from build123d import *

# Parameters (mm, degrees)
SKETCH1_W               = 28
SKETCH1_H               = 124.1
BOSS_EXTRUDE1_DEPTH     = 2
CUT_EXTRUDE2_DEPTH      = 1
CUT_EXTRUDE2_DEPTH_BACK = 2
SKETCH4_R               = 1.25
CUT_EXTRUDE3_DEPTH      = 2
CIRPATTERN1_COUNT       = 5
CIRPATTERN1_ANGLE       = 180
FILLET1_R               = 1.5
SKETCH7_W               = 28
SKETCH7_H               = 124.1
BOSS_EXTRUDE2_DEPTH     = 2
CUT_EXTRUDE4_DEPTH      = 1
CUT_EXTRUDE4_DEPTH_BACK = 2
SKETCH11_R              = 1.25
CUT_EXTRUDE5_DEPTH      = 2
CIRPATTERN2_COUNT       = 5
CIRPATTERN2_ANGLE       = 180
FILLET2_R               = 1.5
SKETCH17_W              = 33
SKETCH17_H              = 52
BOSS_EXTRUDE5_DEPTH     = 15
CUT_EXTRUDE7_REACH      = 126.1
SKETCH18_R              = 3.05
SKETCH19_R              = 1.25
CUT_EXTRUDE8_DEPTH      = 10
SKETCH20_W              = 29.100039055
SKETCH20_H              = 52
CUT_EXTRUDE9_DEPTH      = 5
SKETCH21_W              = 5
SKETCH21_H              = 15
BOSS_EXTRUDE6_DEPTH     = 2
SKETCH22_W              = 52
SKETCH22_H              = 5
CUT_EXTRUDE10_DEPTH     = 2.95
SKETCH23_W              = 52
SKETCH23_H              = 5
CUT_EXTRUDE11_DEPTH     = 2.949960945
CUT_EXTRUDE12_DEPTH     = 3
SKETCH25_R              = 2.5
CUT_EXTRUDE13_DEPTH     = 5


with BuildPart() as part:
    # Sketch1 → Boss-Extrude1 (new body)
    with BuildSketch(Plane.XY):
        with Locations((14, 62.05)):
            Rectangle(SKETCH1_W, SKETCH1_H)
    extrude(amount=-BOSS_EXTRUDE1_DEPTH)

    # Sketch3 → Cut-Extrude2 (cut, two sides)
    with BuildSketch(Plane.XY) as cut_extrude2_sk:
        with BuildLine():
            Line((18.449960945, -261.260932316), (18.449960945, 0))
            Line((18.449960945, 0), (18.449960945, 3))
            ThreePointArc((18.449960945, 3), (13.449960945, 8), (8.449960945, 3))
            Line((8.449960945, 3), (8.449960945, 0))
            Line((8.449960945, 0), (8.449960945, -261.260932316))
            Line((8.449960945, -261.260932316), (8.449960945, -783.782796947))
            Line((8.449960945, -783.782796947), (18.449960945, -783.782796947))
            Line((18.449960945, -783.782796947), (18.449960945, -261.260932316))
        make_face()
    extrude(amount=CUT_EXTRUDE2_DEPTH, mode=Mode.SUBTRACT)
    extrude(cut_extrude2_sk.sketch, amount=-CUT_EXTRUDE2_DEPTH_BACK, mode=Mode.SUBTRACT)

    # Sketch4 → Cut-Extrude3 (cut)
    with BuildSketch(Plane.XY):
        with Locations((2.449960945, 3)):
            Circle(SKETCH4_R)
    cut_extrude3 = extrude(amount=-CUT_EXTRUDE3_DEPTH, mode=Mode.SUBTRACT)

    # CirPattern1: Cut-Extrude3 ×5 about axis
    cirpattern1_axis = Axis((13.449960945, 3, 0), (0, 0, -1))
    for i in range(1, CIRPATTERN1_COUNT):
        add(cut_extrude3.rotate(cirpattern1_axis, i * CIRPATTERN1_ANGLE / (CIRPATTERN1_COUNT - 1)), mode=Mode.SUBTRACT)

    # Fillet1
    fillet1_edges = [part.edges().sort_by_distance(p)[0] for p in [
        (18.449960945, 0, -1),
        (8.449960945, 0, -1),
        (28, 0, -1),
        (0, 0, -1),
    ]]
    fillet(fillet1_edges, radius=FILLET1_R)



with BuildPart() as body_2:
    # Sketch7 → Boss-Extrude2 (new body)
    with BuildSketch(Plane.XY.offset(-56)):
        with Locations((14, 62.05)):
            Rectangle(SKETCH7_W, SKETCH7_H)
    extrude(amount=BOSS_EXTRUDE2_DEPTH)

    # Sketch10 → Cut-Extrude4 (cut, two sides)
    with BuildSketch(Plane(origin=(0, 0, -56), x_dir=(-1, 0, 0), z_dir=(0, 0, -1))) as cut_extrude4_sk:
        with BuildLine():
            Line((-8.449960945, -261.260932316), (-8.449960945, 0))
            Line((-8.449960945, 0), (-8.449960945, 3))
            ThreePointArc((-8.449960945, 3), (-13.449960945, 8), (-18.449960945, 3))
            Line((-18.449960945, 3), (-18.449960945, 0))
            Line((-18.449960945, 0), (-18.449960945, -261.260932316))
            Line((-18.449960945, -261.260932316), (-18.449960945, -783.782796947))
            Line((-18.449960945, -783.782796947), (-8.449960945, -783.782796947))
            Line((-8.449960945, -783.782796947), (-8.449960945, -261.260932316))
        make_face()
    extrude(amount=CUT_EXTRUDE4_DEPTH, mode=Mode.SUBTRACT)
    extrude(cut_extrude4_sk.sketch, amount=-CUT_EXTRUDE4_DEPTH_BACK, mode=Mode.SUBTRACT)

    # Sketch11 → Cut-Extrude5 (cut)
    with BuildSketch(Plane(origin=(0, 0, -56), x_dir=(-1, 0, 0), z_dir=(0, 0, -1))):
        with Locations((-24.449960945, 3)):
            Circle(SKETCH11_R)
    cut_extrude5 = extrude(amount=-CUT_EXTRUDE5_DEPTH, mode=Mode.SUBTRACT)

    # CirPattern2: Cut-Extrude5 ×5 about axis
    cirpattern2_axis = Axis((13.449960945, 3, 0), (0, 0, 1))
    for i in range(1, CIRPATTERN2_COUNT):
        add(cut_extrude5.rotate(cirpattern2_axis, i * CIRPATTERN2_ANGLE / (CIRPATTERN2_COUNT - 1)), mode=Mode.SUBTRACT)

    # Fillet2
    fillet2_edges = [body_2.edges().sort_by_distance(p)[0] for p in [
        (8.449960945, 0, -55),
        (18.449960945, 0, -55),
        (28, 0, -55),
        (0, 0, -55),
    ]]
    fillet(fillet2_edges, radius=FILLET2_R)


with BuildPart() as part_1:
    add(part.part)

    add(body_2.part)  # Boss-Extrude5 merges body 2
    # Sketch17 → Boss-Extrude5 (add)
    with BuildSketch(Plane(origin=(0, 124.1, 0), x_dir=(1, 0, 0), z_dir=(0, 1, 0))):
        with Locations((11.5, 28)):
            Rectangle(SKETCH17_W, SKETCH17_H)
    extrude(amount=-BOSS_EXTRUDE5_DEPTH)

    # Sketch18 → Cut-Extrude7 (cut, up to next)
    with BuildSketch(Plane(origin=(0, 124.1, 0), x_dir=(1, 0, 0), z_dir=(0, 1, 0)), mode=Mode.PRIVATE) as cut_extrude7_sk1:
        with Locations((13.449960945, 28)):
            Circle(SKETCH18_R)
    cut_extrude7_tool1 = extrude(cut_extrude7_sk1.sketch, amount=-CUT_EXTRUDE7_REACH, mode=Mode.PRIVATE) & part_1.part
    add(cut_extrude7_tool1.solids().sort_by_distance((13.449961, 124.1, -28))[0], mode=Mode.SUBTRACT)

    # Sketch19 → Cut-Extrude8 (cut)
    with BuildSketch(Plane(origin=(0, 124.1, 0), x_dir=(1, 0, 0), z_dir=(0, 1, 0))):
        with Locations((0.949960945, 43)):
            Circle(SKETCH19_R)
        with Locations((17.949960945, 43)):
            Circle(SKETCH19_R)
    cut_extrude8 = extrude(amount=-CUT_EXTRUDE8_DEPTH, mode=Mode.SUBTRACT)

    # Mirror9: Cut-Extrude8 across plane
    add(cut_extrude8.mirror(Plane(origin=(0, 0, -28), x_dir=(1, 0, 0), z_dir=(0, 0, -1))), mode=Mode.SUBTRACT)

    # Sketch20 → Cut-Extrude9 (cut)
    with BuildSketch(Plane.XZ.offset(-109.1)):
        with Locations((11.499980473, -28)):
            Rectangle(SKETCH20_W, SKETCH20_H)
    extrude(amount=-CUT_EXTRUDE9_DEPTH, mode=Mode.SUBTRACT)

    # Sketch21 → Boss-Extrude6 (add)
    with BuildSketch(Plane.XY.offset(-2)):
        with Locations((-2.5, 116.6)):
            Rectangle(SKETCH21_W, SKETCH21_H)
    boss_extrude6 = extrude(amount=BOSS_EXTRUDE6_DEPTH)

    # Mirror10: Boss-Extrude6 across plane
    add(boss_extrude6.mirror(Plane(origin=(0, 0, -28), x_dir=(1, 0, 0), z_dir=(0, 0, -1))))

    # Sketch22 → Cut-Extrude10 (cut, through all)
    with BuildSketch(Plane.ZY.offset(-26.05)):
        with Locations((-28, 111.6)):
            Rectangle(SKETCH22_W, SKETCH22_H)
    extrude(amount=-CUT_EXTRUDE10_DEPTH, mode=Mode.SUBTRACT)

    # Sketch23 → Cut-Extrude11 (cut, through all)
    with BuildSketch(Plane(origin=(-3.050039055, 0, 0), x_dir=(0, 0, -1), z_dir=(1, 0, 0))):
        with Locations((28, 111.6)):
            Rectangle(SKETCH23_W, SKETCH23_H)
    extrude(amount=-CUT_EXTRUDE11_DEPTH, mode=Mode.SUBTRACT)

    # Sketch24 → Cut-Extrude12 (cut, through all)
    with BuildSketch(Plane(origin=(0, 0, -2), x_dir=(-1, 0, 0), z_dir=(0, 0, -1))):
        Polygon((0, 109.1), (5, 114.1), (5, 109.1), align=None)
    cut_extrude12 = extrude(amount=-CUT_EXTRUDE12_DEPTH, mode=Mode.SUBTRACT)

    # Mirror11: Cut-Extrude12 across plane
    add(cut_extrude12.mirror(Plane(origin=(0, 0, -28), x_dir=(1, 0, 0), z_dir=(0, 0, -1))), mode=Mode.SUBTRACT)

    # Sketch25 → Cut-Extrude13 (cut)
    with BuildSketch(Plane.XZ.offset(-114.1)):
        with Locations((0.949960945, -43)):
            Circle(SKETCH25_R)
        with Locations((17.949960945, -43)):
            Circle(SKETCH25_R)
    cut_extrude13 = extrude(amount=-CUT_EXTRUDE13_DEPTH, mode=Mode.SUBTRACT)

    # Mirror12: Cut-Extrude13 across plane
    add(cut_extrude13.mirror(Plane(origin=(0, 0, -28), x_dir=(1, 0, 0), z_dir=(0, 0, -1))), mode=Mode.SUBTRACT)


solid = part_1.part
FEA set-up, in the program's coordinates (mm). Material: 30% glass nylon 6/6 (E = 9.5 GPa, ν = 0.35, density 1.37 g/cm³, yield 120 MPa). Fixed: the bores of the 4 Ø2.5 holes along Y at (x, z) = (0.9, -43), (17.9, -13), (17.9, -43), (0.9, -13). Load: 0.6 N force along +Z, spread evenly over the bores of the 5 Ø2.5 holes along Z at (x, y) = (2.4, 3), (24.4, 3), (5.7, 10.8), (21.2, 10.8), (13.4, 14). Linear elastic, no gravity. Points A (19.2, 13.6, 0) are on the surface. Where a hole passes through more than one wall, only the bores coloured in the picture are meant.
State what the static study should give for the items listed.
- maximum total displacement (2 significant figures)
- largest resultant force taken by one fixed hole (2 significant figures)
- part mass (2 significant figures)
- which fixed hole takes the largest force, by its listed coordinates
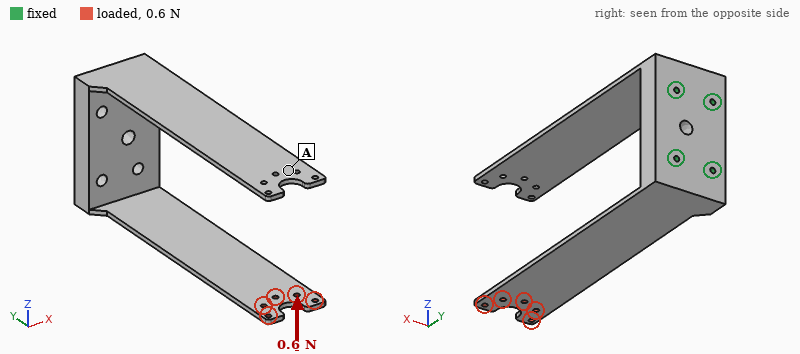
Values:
1.5 mm
1.9 N
41 g
(17.9, -13)
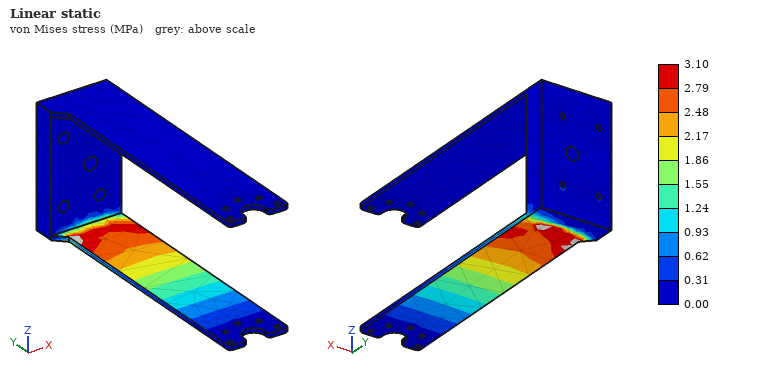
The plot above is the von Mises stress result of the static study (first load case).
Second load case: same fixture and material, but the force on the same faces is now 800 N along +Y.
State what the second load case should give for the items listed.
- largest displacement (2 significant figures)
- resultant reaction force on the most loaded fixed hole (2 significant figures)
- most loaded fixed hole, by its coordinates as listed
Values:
0.86 mm
730 N
(17.9, -43)
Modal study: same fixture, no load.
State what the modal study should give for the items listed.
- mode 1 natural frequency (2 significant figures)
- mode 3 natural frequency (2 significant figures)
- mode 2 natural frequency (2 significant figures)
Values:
70 Hz
430 Hz
70 Hz
